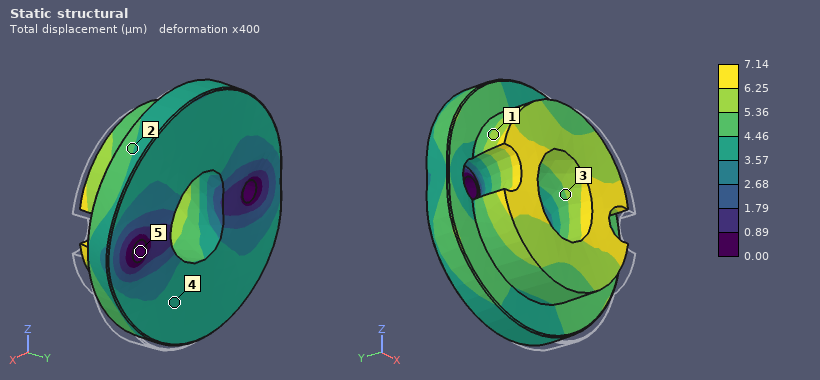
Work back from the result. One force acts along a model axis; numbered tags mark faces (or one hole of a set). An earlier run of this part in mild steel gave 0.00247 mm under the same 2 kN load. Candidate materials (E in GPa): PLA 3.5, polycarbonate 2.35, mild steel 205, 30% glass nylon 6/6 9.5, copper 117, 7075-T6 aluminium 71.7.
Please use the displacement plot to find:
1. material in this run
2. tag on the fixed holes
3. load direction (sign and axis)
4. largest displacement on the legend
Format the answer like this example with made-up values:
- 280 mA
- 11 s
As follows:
- 7075-T6 aluminium
- 5
- -X
- 7.14 µm
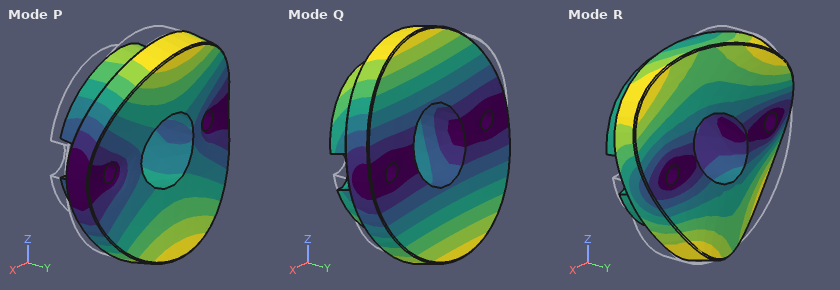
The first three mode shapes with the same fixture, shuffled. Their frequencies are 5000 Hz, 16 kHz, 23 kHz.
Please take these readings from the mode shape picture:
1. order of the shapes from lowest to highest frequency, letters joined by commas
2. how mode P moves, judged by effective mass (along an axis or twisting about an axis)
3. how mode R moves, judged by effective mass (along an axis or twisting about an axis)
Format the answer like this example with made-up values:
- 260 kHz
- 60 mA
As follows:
- Q, P, R
- along Y
- twisting about Y
